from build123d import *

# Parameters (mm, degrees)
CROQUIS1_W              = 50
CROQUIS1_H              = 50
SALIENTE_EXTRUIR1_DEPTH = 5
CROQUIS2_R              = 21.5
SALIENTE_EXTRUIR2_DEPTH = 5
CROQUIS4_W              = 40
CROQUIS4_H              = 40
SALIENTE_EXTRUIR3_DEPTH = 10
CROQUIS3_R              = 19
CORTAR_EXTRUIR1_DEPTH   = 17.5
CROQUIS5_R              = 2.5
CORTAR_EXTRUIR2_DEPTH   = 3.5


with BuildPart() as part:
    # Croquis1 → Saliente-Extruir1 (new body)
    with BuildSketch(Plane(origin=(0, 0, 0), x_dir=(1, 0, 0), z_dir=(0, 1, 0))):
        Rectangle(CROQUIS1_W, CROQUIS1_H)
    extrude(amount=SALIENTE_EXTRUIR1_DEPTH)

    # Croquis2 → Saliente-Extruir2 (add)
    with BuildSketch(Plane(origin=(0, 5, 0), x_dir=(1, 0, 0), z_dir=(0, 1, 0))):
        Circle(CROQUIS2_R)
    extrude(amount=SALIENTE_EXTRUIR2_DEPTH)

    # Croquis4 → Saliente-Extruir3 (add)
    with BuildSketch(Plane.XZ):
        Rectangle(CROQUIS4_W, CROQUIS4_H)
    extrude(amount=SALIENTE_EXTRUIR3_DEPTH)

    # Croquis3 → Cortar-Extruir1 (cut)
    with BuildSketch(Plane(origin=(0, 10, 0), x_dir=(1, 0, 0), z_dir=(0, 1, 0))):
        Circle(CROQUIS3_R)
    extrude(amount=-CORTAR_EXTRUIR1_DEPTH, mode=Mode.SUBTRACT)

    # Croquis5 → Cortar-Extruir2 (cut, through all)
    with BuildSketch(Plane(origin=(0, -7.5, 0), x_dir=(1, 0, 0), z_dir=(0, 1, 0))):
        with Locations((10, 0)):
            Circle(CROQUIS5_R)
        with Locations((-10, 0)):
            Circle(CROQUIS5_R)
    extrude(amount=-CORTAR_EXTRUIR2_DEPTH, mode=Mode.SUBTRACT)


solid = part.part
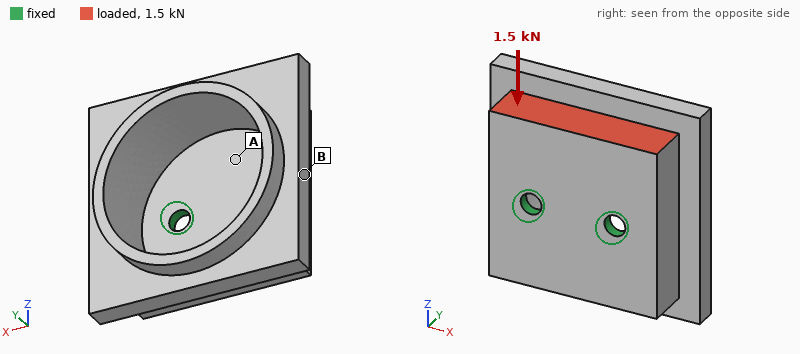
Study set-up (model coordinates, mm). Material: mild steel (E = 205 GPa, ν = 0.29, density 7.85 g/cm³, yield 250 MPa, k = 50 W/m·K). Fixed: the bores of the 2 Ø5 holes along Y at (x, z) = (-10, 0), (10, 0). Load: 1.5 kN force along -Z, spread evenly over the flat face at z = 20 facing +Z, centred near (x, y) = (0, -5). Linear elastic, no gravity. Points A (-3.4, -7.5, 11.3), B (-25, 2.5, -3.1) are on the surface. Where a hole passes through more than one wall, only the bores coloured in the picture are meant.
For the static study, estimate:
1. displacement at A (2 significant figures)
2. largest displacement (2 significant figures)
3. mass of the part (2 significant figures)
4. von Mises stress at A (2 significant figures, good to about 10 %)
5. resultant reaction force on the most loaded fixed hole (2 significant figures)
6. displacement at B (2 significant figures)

8.7 µm
31 µm
120 g
26 MPa
760 N
13 µm
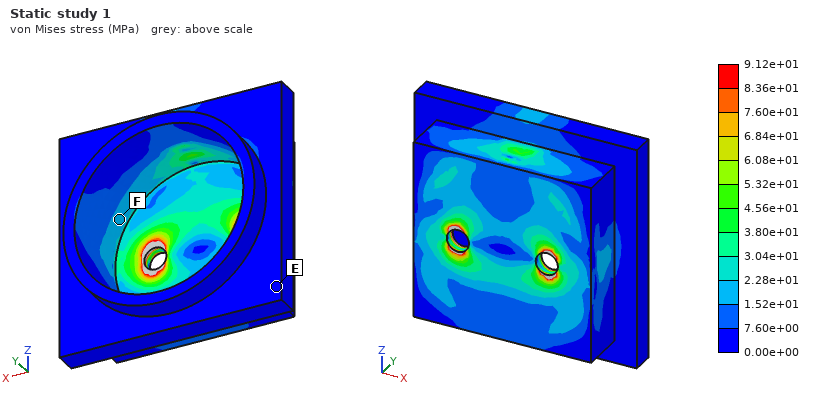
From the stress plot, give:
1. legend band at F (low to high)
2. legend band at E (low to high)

1.52e+01 to 2.28e+01 MPa
0.00e+00 to 7.60e+00 MPa
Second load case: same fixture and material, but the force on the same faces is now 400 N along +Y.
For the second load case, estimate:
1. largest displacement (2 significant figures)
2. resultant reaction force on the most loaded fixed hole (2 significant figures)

42 µm
210 N
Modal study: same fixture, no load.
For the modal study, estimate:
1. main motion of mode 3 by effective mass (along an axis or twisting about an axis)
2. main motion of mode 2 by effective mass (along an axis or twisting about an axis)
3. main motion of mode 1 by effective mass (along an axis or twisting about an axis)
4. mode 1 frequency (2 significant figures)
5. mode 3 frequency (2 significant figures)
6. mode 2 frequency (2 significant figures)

along Y
along X
along Z
1900 Hz
5500 Hz
4100 Hz
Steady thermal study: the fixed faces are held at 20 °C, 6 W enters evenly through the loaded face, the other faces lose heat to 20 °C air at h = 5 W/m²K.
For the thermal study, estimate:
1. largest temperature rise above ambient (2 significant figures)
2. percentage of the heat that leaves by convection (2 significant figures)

17 K
6.3 %
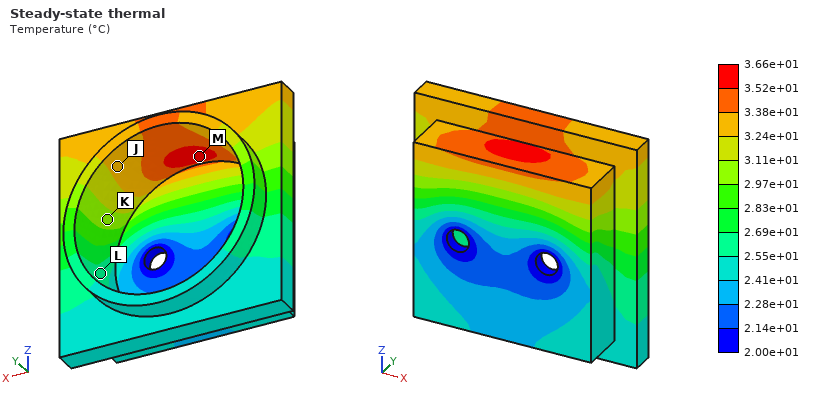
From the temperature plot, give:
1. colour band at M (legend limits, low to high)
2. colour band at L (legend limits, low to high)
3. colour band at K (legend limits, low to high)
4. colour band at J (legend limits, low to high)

3.52e+01 to 3.66e+01 °C
2.55e+01 to 2.69e+01 °C
2.97e+01 to 3.11e+01 °C
3.24e+01 to 3.38e+01 °C
